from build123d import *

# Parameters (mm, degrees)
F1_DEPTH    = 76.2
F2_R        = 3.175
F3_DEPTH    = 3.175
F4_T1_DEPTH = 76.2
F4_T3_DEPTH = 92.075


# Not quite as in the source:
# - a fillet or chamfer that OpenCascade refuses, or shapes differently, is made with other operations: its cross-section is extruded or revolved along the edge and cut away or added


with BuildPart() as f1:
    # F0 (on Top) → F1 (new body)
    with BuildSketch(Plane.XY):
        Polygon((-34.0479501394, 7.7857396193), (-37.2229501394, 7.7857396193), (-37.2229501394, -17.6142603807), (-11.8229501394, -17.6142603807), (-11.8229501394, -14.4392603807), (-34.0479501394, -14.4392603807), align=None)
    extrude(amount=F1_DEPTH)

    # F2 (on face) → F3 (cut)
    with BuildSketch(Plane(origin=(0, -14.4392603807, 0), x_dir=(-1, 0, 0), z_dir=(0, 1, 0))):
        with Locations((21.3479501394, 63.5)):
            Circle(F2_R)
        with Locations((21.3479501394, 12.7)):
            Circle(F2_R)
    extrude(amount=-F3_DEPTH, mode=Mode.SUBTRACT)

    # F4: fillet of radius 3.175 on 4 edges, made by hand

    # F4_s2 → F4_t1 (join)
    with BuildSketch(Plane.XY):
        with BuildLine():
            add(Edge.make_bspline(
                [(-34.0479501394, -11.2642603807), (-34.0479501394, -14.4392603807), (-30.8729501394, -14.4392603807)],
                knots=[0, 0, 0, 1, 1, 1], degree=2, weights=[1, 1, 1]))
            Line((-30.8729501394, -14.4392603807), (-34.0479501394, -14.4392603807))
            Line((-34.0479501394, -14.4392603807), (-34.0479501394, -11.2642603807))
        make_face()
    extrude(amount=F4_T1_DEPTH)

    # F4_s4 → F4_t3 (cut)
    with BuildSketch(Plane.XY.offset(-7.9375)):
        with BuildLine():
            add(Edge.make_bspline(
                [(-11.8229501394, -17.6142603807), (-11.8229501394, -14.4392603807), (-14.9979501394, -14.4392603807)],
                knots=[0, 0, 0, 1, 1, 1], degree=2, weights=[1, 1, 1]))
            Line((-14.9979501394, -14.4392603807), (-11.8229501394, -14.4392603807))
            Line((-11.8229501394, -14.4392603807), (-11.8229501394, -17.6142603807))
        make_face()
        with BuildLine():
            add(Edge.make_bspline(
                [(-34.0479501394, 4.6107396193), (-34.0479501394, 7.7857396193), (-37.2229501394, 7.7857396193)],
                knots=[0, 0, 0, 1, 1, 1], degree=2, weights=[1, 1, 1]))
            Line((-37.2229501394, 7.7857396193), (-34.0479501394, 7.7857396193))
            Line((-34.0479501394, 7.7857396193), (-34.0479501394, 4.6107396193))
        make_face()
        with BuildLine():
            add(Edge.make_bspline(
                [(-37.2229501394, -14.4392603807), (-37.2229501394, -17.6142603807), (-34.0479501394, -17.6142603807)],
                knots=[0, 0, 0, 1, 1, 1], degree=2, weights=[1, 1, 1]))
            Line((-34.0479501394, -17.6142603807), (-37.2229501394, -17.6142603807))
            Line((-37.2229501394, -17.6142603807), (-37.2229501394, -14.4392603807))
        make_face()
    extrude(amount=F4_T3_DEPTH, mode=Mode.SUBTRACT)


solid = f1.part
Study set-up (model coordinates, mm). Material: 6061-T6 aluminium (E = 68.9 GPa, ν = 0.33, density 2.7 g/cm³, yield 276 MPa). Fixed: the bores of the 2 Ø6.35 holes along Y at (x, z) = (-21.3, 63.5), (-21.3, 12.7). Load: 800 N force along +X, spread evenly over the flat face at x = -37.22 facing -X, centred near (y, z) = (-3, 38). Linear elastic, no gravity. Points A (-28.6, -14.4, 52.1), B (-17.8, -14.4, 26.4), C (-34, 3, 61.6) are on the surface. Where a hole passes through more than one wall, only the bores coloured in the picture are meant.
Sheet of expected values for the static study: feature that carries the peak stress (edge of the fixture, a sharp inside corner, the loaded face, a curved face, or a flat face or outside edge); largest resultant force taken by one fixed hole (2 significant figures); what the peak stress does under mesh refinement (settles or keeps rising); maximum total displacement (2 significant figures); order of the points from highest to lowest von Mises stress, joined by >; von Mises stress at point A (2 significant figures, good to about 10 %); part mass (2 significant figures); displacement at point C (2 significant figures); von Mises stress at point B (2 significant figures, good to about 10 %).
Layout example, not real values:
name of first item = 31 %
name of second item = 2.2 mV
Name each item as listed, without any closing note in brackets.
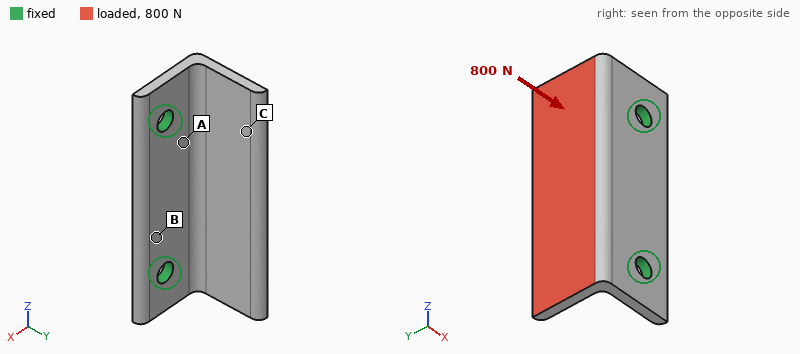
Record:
feature that carries the peak stress = edge of the fixture
largest resultant force taken by one fixed hole = 410 N
what the peak stress does under mesh refinement = keeps rising
maximum total displacement = 0.30 mm
order of the points from highest to lowest von Mises stress, joined by > = A > B > C
von Mises stress at point A = 66 MPa
part mass = 30 g
displacement at point C = 0.23 mm
von Mises stress at point B = 30 MPa
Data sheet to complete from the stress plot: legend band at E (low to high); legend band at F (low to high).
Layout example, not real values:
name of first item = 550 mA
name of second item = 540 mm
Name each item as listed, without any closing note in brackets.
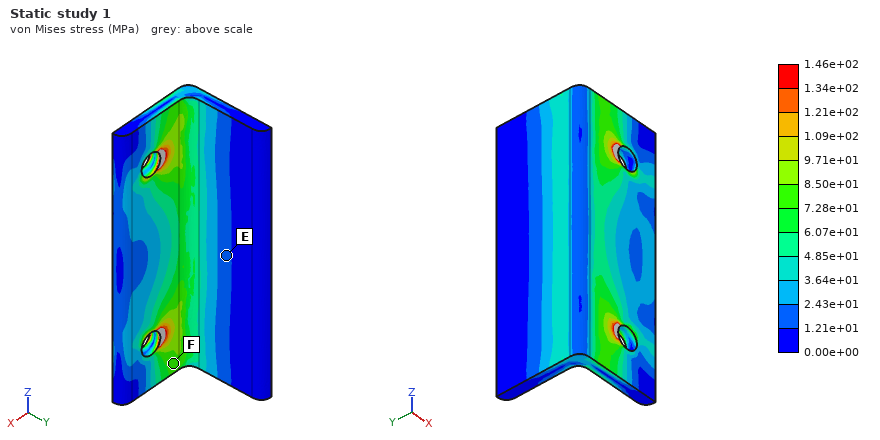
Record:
legend band at E = 1.21e+01 to 2.43e+01 MPa
legend band at F = 7.28e+01 to 8.50e+01 MPa
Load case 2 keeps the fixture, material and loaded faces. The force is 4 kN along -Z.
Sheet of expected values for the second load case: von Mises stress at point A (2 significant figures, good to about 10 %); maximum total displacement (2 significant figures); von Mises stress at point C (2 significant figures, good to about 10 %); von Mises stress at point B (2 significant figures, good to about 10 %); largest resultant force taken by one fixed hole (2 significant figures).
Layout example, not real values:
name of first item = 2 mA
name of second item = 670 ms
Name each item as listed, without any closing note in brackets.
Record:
von Mises stress at point A = 83 MPa
maximum total displacement = 0.21 mm
von Mises stress at point C = 21 MPa
von Mises stress at point B = 20 MPa
largest resultant force taken by one fixed hole = 2.5 kN
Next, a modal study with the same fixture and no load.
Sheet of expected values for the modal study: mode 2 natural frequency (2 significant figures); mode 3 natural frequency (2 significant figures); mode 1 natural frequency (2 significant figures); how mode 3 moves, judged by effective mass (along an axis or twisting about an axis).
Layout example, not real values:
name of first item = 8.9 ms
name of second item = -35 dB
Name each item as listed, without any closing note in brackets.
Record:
mode 2 natural frequency = 3800 Hz
mode 3 natural frequency = 6800 Hz
mode 1 natural frequency = 2500 Hz
how mode 3 moves, judged by effective mass = along Y
